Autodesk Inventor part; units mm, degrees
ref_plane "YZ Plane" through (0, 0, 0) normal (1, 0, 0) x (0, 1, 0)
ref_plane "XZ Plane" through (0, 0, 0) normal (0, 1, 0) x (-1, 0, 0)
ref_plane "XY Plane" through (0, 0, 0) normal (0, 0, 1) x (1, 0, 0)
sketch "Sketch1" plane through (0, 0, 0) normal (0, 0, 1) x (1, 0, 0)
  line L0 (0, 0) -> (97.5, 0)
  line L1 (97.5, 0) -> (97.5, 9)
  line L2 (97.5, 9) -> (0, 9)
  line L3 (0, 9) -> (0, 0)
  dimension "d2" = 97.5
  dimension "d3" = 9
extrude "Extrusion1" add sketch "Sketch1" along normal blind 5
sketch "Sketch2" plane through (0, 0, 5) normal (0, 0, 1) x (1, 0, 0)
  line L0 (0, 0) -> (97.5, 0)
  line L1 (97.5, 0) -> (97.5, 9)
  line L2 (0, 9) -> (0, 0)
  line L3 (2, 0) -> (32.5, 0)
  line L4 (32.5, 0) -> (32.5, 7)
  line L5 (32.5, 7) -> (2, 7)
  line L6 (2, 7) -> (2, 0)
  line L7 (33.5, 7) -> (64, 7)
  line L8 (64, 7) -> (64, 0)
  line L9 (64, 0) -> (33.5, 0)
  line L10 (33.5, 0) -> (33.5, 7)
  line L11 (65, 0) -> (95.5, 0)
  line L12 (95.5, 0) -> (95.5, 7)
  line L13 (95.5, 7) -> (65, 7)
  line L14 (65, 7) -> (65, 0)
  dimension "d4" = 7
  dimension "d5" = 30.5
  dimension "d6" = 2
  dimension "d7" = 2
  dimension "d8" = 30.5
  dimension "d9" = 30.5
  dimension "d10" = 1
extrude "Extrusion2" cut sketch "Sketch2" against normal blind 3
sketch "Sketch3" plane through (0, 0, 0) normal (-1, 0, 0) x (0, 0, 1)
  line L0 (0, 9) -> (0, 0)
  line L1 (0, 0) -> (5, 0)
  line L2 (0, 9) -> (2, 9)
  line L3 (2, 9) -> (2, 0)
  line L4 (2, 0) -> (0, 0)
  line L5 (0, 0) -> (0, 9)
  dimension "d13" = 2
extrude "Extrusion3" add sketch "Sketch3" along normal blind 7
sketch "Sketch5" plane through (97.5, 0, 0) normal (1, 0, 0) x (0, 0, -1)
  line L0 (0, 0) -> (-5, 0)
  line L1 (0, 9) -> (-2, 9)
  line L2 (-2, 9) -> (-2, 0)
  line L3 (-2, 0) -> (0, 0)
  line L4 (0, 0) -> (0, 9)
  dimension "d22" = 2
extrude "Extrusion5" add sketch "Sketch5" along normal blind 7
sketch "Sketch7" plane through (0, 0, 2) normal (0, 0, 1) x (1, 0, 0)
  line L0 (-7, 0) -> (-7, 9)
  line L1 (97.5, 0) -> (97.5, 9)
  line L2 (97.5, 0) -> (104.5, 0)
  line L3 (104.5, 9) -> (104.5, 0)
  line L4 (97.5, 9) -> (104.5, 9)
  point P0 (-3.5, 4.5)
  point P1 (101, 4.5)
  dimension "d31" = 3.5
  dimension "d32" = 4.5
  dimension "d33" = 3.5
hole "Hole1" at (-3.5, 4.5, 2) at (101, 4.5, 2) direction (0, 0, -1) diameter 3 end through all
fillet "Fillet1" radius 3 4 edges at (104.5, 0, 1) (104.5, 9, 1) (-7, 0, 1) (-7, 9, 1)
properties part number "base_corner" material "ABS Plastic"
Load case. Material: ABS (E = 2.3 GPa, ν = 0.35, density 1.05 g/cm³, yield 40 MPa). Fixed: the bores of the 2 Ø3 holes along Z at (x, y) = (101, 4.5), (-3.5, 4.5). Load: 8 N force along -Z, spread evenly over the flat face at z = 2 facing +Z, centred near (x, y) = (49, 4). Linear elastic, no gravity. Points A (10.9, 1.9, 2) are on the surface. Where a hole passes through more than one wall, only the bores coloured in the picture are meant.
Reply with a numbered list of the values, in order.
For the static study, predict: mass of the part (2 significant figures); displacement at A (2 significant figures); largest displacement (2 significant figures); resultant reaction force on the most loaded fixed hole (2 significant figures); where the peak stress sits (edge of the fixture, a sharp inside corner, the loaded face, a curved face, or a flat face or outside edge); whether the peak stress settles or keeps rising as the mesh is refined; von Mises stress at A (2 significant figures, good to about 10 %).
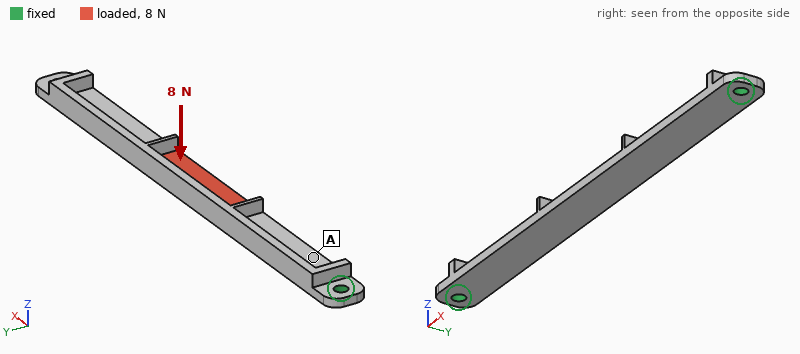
1. 2.8 g
2. 0.26 mm
3. 1.1 mm
4. 11 N
5. edge of the fixture
6. keeps rising
7. 2.1 MPa
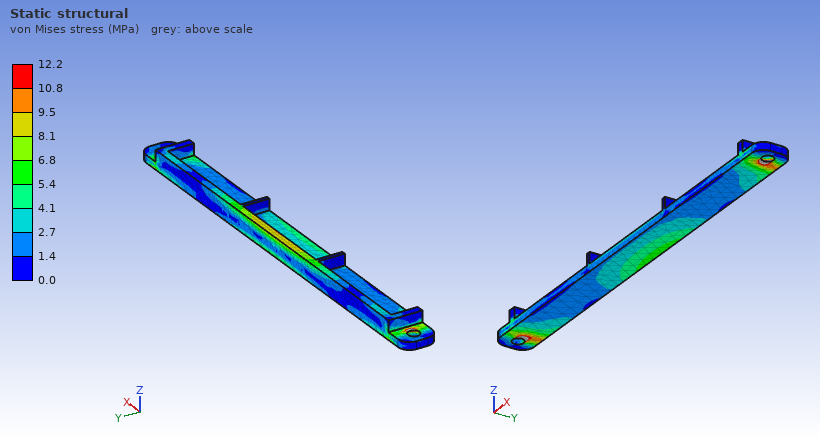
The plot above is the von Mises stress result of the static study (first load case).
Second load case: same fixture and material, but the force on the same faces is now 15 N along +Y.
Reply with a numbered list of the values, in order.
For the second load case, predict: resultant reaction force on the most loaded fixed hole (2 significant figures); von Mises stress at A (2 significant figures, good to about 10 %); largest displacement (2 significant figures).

1. 8.1 N
2. 2.5 MPa
3. 0.48 mm
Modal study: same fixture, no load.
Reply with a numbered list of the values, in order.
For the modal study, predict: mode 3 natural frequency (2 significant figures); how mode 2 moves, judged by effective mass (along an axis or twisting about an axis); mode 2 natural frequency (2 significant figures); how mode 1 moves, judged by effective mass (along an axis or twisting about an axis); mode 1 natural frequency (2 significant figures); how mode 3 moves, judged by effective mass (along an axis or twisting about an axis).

1. 1200 Hz
2. along Y
3. 980 Hz
4. along Z
5. 420 Hz
6. twisting about Y
